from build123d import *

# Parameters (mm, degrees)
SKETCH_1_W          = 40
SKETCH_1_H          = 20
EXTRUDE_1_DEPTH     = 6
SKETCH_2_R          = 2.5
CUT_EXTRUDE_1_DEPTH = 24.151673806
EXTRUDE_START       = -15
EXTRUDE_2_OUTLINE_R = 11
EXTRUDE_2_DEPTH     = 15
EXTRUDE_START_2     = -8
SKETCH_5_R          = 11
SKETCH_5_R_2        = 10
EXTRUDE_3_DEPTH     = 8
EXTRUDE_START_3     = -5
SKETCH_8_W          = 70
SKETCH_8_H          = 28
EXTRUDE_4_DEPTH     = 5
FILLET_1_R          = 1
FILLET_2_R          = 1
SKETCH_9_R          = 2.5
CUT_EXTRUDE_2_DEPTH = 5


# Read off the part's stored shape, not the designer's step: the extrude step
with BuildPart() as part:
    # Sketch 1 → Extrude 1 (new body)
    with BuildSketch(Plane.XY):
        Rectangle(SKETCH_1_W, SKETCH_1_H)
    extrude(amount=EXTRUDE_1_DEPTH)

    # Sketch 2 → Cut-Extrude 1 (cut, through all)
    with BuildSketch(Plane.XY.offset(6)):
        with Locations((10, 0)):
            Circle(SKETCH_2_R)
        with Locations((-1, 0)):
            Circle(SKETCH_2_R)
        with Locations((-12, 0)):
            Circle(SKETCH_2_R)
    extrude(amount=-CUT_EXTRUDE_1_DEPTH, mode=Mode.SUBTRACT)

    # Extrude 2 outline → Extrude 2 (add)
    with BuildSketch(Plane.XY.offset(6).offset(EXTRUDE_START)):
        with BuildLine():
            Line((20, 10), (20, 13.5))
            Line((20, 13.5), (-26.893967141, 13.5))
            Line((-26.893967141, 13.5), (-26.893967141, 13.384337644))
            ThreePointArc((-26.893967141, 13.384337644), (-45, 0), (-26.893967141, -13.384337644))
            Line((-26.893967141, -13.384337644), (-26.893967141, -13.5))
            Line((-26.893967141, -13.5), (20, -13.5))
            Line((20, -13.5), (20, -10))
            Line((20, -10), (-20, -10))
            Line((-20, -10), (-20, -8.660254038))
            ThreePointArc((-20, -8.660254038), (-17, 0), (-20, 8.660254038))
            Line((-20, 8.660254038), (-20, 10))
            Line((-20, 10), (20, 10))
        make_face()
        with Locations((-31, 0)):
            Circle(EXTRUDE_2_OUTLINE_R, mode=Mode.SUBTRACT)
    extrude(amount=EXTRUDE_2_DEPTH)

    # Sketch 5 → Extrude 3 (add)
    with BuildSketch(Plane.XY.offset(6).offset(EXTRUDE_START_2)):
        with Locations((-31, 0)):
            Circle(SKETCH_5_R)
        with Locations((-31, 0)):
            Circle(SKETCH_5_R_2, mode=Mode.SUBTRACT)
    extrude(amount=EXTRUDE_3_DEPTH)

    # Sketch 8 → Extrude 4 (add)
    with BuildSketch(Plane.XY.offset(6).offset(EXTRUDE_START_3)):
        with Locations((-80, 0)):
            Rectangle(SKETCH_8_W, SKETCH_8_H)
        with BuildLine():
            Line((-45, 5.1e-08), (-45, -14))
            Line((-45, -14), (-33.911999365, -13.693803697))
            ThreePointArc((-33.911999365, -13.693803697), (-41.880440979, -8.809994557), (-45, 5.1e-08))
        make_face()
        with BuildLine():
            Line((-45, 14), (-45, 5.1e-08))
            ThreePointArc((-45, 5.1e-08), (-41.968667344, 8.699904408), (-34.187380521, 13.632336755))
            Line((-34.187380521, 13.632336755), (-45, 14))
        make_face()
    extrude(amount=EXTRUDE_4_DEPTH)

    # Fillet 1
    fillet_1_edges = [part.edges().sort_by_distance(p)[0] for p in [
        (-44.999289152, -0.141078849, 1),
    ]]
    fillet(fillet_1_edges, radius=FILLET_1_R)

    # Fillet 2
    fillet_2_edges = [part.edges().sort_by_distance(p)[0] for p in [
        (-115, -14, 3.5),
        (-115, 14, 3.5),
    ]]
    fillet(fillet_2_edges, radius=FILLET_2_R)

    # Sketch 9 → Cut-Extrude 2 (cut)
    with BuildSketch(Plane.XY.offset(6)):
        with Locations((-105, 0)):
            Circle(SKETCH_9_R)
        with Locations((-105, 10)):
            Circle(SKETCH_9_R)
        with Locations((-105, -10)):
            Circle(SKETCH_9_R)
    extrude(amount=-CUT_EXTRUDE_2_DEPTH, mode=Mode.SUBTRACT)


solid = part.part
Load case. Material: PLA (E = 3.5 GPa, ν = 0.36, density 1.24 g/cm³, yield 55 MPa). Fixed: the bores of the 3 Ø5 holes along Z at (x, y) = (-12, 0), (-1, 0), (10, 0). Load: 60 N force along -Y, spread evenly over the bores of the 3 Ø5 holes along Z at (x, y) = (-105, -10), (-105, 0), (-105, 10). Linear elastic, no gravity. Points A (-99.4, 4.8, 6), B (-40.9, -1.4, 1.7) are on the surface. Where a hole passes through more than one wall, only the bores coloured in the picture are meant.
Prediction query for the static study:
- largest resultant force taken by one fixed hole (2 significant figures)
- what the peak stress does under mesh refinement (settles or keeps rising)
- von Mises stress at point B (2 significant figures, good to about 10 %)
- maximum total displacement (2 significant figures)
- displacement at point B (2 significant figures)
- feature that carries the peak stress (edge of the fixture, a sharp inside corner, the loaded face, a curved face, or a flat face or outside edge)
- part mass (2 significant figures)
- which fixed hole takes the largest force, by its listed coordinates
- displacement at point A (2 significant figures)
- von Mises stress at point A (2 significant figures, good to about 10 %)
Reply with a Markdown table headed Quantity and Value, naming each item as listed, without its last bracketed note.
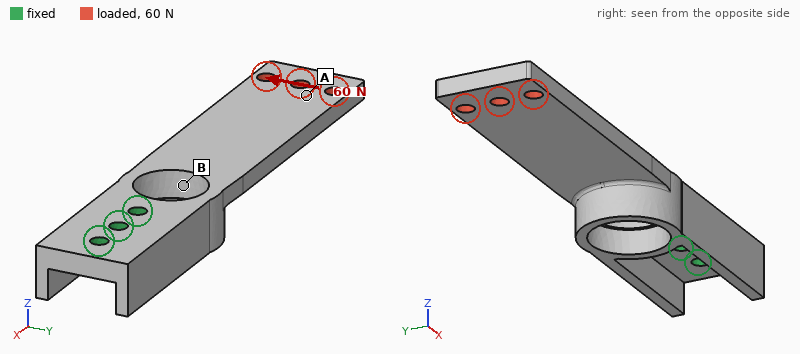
| Quantity | Value |
|---|---|
| largest resultant force taken by one fixed hole | 280 N |
| what the peak stress does under mesh refinement | keeps rising |
| von Mises stress at point B | 2.7 MPa |
| maximum total displacement | 0.79 mm |
| displacement at point B | 0.14 mm |
| feature that carries the peak stress | edge of the fixture |
| part mass | 28 g |
| which fixed hole takes the largest force, by its listed coordinates | (-12, 0) |
| displacement at point A | 0.62 mm |
| von Mises stress at point A | 0.79 MPa |
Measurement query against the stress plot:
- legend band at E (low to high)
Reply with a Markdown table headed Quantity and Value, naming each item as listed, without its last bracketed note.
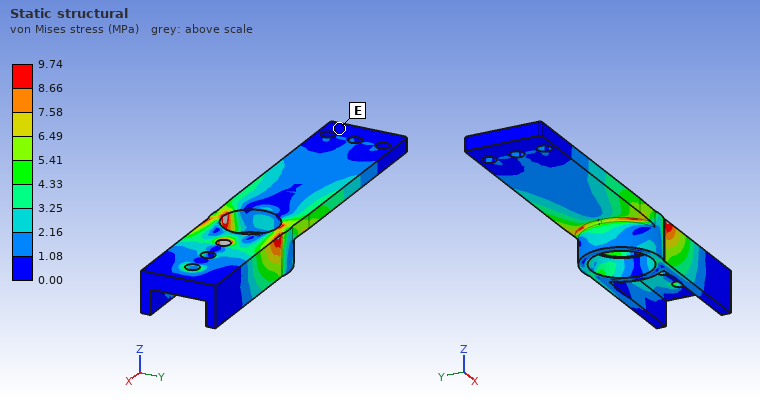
| Quantity | Value |
|---|---|
| legend band at E | 0.00 to 1.08 MPa |
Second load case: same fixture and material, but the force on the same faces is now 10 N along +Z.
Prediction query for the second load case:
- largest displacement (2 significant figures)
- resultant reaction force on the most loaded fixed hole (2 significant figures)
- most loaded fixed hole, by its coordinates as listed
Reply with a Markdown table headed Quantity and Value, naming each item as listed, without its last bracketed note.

| Quantity | Value |
|---|---|
| largest displacement | 1.5 mm |
| resultant reaction force on the most loaded fixed hole | 47 N |
| most loaded fixed hole, by its coordinates as listed | (-12, 0) |
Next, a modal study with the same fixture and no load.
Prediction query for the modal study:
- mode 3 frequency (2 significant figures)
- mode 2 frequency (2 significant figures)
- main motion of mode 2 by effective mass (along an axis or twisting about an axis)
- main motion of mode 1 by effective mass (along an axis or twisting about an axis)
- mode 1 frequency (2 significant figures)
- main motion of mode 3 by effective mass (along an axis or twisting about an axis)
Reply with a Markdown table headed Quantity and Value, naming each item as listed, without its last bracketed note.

| Quantity | Value |
|---|---|
| mode 3 frequency | 1000 Hz |
| mode 2 frequency | 600 Hz |
| main motion of mode 2 by effective mass | along Y |
| main motion of mode 1 by effective mass | along Z |
| mode 1 frequency | 200 Hz |
| main motion of mode 3 by effective mass | twisting about X |
